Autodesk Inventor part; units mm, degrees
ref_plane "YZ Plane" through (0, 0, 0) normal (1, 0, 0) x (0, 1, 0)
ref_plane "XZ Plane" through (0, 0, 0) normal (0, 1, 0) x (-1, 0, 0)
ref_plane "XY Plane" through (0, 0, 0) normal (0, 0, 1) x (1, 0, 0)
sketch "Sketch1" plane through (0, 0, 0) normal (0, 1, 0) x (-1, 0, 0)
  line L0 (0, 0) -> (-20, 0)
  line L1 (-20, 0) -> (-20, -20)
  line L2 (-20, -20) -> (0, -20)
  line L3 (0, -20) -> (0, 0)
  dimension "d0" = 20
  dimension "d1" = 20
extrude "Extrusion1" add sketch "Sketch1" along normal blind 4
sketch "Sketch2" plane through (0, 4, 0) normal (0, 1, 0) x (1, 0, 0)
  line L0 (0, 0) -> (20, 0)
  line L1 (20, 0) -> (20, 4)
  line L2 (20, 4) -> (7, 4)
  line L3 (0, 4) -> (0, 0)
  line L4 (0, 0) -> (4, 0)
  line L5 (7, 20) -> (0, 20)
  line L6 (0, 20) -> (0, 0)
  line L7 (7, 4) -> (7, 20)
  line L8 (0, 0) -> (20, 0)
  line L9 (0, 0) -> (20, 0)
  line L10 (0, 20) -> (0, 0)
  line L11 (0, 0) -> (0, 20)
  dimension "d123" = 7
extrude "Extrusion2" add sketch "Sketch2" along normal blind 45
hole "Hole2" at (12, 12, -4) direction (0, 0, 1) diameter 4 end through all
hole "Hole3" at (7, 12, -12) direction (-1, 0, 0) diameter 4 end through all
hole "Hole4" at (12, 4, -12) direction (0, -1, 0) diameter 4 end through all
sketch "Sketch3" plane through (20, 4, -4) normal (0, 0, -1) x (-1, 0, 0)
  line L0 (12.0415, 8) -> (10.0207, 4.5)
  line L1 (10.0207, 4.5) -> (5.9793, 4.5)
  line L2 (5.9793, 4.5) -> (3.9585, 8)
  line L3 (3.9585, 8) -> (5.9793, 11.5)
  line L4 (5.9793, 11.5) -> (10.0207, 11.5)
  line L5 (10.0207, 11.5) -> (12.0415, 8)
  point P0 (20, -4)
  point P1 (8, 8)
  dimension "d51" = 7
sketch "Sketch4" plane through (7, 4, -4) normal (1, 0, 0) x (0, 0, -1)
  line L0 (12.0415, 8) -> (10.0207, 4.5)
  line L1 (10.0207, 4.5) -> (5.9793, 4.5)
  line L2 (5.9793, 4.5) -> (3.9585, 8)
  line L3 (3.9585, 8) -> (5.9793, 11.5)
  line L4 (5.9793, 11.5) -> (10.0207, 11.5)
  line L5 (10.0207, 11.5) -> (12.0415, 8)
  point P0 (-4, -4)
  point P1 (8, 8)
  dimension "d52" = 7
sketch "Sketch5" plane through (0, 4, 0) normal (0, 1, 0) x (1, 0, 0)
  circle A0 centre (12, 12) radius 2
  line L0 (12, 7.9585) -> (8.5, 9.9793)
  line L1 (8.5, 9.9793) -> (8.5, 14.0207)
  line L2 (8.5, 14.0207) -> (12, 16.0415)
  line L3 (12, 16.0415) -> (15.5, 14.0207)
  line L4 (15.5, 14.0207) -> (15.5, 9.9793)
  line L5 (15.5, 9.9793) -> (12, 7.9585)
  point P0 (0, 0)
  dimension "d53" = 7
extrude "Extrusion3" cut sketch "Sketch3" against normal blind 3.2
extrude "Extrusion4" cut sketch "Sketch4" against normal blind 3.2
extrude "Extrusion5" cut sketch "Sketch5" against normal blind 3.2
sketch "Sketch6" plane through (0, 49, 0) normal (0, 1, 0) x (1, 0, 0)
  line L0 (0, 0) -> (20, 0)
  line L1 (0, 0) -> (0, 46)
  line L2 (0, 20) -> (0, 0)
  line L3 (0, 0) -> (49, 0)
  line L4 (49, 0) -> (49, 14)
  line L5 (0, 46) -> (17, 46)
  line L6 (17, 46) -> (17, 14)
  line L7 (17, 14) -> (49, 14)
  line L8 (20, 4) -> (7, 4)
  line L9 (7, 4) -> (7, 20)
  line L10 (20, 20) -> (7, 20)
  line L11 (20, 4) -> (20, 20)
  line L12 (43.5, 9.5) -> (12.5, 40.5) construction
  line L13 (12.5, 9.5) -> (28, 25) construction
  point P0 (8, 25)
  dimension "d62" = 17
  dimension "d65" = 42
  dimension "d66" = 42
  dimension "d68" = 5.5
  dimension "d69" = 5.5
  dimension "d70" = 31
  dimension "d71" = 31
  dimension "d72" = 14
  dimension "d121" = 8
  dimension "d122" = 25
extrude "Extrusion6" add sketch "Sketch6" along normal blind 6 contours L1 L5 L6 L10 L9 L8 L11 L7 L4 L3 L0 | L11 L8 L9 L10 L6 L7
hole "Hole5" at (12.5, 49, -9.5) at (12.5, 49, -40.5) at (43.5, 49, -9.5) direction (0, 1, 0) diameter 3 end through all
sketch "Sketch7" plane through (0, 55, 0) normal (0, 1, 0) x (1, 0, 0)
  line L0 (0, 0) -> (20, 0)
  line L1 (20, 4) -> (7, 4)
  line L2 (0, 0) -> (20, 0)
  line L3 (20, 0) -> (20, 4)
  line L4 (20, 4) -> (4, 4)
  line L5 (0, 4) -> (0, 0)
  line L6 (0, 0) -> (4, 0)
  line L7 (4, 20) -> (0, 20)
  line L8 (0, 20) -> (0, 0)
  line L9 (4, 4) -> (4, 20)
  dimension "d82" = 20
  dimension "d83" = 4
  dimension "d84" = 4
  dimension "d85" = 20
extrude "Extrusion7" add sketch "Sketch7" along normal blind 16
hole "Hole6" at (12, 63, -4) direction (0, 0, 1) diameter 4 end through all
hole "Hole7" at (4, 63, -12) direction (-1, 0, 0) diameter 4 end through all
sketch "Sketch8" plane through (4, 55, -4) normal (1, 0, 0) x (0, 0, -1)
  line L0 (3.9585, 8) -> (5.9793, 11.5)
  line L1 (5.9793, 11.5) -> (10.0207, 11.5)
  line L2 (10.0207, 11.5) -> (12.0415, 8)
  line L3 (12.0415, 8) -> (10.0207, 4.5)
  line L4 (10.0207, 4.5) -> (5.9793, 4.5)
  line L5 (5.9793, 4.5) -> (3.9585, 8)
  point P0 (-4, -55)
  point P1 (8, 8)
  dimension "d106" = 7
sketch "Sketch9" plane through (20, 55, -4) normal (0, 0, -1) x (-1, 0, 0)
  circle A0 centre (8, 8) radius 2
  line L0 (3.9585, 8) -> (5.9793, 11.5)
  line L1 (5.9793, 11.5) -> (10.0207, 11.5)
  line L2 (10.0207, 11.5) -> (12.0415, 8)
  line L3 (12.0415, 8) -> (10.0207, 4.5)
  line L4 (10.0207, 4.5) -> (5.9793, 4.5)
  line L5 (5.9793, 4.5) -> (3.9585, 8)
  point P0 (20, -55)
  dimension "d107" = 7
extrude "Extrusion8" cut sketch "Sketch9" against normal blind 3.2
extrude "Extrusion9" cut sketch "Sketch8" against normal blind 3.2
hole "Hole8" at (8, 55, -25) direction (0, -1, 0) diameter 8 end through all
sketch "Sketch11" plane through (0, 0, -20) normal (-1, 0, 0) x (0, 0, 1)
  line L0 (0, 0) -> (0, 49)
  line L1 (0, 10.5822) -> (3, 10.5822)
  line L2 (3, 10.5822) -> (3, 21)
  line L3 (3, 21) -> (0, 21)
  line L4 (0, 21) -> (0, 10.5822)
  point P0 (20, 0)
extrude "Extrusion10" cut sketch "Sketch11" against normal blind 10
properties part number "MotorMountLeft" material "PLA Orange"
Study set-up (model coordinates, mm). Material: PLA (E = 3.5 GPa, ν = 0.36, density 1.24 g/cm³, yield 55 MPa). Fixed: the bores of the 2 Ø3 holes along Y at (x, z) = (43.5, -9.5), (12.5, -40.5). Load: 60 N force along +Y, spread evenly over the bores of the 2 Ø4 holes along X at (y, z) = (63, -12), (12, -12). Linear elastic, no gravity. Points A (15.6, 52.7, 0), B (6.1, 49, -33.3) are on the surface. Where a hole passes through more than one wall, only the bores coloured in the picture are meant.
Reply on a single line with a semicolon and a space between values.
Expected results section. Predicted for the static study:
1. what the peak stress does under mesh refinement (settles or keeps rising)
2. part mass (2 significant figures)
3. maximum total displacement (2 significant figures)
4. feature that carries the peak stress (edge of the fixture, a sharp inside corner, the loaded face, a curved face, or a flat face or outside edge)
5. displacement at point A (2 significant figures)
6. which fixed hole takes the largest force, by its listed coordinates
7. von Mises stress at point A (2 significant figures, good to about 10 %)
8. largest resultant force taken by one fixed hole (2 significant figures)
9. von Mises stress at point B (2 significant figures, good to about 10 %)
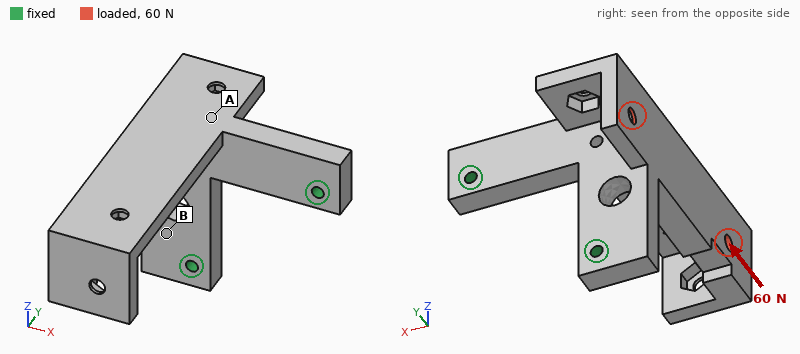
keeps rising; 23 g; 1.0 mm; edge of the fixture; 0.29 mm; (12.5, -40.5); 2.6 MPa; 43 N; 7.5 MPa
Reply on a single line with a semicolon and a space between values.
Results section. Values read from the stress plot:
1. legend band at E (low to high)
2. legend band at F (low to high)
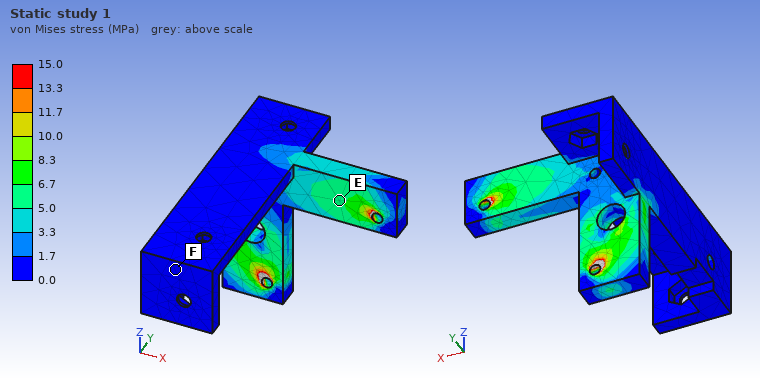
5.0 to 6.7 MPa; 0.0 to 1.7 MPa
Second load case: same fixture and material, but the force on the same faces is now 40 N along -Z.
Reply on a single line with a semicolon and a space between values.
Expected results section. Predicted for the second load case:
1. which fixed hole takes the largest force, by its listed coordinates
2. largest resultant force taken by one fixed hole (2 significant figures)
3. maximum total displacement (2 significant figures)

(12.5, -40.5); 48 N; 1.0 mm
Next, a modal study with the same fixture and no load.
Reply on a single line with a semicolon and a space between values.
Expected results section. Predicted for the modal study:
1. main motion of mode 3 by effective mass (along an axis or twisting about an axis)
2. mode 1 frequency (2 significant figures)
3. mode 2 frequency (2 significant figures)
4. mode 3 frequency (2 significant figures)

along Y; 280 Hz; 640 Hz; 1100 Hz
